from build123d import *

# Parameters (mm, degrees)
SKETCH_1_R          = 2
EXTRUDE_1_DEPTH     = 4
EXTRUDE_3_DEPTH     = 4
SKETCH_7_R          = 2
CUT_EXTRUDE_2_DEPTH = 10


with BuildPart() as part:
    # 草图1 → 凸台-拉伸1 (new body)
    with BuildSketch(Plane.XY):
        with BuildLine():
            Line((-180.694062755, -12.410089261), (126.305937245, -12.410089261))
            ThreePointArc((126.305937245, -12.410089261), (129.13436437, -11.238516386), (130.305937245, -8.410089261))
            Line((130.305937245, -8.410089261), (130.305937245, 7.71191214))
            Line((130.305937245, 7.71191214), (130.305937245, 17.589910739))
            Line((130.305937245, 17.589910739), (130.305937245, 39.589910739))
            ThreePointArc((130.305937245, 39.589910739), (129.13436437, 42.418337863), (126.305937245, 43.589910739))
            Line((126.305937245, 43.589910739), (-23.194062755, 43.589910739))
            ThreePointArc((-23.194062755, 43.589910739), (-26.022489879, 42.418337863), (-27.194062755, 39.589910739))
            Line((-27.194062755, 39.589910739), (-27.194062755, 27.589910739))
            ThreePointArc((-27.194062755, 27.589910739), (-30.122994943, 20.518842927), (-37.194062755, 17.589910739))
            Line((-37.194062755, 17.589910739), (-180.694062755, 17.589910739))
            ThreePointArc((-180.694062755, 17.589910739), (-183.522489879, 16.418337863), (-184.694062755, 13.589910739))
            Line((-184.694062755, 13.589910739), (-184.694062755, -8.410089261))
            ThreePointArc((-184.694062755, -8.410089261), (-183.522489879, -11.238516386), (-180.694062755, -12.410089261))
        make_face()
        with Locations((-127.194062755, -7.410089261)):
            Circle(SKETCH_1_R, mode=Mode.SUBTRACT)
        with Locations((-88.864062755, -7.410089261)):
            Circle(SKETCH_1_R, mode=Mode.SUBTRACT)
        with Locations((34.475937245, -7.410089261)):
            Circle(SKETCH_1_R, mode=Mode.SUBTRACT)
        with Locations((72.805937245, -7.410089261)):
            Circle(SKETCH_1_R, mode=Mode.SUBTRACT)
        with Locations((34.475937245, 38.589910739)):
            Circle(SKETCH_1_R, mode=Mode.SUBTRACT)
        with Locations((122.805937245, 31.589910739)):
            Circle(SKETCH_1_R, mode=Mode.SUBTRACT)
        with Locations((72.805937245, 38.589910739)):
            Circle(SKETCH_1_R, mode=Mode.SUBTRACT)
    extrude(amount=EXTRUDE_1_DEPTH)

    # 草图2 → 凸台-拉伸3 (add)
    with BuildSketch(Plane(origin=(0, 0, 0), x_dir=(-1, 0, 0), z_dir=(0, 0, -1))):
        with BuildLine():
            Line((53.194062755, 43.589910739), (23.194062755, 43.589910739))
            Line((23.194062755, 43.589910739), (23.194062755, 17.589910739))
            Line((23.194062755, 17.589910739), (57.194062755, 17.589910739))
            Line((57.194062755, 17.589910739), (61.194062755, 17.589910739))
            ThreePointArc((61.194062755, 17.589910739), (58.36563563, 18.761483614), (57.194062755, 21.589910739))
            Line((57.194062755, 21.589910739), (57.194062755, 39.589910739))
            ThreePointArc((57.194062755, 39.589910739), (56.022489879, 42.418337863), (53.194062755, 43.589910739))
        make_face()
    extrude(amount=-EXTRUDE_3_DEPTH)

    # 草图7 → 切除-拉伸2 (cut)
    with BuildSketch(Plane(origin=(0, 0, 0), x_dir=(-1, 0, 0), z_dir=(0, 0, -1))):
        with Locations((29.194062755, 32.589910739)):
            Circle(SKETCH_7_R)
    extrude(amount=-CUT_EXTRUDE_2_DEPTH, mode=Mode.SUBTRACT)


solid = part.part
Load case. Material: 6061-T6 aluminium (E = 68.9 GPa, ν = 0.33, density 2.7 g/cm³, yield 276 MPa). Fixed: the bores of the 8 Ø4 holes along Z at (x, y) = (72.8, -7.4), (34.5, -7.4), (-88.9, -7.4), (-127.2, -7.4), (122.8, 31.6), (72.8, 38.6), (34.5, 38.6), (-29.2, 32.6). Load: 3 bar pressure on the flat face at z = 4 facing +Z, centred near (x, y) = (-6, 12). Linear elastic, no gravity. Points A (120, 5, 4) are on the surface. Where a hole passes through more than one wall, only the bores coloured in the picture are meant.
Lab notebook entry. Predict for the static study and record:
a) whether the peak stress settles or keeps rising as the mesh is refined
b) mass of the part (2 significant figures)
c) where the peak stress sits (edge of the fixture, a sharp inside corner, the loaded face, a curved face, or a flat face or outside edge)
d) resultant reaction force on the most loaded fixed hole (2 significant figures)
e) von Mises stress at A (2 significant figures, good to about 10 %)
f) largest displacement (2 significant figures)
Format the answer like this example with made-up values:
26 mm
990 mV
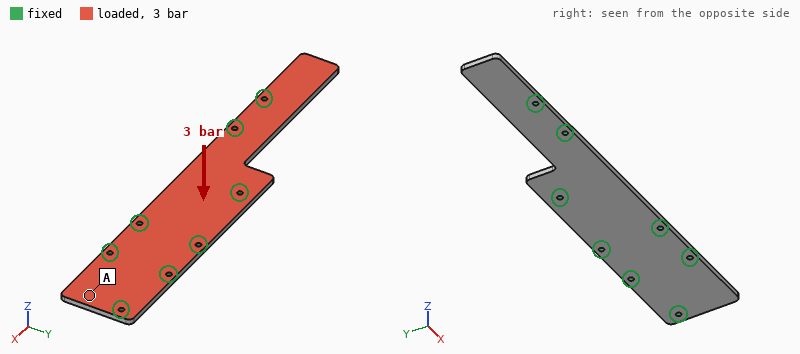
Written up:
keeps rising
150 g
edge of the fixture
880 N
20 MPa
1.4 mm
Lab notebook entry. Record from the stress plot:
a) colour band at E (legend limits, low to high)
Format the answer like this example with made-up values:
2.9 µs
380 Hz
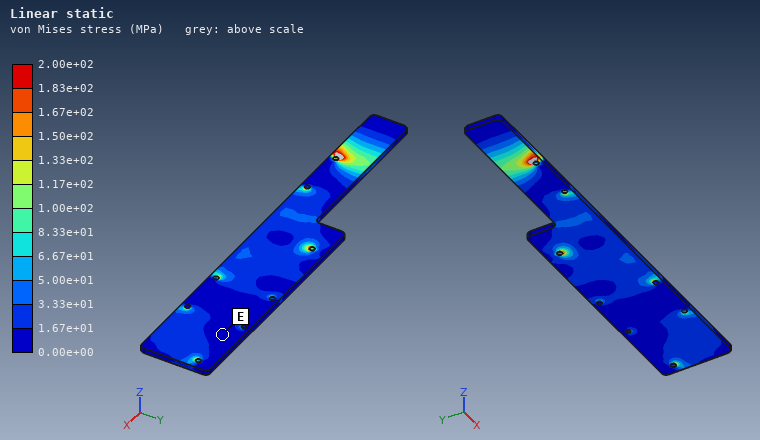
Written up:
0.00e+00 to 1.67e+01 MPa
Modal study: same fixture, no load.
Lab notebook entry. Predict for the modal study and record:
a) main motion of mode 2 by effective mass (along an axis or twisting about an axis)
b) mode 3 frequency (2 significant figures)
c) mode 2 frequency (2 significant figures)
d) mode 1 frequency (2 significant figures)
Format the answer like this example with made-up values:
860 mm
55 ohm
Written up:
along Z
2600 Hz
2200 Hz
910 Hz
